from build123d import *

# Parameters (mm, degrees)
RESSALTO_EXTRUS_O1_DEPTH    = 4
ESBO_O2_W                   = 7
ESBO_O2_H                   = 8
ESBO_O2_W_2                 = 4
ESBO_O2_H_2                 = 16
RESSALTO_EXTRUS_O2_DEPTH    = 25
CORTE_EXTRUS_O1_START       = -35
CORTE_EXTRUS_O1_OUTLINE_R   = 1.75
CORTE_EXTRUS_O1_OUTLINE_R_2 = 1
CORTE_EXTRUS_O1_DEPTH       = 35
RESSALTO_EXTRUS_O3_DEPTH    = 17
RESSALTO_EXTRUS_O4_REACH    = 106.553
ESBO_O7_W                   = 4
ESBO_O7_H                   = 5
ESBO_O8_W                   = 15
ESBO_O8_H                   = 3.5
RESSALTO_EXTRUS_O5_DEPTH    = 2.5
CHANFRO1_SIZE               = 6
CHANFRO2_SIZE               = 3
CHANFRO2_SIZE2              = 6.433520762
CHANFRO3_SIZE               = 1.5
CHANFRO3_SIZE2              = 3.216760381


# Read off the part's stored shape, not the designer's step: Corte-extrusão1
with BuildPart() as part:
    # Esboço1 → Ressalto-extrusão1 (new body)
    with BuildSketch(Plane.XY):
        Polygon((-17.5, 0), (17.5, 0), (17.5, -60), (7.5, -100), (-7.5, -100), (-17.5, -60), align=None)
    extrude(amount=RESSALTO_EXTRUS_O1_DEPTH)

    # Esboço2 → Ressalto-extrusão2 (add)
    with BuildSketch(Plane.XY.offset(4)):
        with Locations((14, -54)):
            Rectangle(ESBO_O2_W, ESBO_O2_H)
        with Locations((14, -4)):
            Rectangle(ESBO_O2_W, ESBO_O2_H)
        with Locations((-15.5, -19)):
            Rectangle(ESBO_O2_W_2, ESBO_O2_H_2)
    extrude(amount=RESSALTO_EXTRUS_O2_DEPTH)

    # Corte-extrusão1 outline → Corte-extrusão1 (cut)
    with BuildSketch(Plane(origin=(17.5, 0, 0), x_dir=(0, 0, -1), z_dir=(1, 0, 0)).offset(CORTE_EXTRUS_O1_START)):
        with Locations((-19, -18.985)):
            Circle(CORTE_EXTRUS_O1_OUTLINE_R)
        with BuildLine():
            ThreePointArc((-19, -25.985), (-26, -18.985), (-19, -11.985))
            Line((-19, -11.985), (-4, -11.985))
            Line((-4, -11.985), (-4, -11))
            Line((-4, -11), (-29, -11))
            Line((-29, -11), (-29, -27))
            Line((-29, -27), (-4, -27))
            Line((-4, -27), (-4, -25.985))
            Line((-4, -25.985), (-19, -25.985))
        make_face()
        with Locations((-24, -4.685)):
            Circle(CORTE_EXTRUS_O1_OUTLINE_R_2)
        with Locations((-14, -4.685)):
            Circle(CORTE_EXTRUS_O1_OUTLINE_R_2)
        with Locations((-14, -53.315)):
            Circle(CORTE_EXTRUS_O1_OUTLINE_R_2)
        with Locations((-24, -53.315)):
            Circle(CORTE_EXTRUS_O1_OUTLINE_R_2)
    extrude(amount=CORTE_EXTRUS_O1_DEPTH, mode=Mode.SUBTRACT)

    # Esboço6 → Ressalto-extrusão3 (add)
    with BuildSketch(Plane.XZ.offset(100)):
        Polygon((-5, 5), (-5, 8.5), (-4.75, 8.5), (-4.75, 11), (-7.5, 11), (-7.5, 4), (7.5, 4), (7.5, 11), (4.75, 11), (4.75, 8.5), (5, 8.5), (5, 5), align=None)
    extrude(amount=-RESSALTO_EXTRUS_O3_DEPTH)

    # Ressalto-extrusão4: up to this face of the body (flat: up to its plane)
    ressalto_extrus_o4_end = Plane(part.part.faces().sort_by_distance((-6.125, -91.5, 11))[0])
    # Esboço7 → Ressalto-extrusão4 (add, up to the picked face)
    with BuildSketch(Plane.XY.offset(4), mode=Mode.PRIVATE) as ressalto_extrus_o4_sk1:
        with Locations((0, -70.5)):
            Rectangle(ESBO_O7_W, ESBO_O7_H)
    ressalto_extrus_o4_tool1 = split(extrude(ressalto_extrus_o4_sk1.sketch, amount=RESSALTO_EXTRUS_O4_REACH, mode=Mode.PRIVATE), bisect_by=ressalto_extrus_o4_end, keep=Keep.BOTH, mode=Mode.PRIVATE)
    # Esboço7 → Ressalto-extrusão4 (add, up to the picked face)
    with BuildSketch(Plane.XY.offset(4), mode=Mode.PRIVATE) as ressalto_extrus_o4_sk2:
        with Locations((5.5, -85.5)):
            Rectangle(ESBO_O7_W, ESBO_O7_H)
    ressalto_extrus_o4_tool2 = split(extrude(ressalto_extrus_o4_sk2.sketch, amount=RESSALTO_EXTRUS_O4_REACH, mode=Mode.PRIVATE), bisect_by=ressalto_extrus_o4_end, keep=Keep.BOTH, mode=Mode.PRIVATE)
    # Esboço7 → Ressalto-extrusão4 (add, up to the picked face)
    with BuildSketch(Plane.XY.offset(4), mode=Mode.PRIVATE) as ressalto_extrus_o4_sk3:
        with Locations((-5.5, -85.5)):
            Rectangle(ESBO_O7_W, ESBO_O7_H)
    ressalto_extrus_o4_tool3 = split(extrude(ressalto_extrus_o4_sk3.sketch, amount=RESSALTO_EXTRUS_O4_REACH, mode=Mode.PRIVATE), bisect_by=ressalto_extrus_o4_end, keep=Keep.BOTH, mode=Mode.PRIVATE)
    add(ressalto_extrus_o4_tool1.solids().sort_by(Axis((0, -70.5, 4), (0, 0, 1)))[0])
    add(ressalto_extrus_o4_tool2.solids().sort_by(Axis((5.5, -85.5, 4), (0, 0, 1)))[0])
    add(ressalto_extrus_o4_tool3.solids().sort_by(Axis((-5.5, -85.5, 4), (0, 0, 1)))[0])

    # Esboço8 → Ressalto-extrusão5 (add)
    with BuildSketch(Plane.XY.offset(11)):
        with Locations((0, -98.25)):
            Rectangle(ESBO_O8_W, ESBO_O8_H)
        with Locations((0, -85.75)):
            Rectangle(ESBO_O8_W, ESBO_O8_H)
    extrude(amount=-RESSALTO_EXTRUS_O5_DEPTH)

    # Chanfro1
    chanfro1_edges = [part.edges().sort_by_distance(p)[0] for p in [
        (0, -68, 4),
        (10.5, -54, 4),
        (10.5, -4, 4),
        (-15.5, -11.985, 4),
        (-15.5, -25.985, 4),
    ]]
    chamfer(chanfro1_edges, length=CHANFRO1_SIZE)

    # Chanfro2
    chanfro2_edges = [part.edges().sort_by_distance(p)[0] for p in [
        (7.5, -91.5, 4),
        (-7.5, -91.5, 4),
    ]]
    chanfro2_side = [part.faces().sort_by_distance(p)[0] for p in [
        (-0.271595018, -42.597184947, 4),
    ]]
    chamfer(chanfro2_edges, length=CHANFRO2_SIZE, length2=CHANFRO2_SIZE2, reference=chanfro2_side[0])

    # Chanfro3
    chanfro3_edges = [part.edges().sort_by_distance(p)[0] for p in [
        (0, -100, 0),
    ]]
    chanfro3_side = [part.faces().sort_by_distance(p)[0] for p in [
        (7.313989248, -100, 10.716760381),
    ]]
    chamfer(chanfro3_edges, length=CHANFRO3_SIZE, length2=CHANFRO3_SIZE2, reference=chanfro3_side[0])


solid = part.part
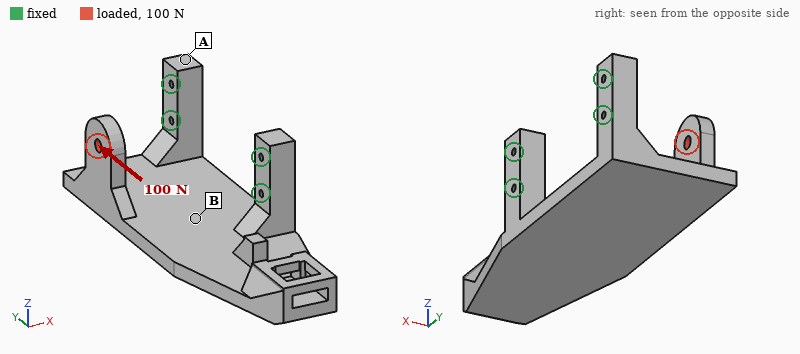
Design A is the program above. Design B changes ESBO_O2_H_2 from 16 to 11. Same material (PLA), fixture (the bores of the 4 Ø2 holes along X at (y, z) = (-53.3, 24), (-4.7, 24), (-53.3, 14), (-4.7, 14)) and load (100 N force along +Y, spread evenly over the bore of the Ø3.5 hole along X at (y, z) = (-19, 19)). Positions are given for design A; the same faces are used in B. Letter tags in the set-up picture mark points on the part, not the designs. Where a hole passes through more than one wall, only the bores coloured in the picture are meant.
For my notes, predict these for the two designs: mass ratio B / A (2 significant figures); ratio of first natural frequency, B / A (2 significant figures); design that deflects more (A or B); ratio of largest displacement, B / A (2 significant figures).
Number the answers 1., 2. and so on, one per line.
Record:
1. 0.99
2. 1.00
3. B
4. 1.1
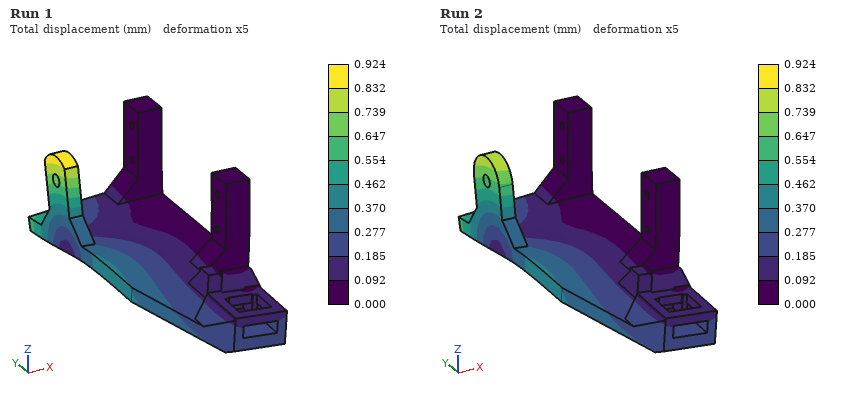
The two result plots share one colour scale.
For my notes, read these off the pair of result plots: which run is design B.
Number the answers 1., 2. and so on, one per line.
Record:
1. Run 1
